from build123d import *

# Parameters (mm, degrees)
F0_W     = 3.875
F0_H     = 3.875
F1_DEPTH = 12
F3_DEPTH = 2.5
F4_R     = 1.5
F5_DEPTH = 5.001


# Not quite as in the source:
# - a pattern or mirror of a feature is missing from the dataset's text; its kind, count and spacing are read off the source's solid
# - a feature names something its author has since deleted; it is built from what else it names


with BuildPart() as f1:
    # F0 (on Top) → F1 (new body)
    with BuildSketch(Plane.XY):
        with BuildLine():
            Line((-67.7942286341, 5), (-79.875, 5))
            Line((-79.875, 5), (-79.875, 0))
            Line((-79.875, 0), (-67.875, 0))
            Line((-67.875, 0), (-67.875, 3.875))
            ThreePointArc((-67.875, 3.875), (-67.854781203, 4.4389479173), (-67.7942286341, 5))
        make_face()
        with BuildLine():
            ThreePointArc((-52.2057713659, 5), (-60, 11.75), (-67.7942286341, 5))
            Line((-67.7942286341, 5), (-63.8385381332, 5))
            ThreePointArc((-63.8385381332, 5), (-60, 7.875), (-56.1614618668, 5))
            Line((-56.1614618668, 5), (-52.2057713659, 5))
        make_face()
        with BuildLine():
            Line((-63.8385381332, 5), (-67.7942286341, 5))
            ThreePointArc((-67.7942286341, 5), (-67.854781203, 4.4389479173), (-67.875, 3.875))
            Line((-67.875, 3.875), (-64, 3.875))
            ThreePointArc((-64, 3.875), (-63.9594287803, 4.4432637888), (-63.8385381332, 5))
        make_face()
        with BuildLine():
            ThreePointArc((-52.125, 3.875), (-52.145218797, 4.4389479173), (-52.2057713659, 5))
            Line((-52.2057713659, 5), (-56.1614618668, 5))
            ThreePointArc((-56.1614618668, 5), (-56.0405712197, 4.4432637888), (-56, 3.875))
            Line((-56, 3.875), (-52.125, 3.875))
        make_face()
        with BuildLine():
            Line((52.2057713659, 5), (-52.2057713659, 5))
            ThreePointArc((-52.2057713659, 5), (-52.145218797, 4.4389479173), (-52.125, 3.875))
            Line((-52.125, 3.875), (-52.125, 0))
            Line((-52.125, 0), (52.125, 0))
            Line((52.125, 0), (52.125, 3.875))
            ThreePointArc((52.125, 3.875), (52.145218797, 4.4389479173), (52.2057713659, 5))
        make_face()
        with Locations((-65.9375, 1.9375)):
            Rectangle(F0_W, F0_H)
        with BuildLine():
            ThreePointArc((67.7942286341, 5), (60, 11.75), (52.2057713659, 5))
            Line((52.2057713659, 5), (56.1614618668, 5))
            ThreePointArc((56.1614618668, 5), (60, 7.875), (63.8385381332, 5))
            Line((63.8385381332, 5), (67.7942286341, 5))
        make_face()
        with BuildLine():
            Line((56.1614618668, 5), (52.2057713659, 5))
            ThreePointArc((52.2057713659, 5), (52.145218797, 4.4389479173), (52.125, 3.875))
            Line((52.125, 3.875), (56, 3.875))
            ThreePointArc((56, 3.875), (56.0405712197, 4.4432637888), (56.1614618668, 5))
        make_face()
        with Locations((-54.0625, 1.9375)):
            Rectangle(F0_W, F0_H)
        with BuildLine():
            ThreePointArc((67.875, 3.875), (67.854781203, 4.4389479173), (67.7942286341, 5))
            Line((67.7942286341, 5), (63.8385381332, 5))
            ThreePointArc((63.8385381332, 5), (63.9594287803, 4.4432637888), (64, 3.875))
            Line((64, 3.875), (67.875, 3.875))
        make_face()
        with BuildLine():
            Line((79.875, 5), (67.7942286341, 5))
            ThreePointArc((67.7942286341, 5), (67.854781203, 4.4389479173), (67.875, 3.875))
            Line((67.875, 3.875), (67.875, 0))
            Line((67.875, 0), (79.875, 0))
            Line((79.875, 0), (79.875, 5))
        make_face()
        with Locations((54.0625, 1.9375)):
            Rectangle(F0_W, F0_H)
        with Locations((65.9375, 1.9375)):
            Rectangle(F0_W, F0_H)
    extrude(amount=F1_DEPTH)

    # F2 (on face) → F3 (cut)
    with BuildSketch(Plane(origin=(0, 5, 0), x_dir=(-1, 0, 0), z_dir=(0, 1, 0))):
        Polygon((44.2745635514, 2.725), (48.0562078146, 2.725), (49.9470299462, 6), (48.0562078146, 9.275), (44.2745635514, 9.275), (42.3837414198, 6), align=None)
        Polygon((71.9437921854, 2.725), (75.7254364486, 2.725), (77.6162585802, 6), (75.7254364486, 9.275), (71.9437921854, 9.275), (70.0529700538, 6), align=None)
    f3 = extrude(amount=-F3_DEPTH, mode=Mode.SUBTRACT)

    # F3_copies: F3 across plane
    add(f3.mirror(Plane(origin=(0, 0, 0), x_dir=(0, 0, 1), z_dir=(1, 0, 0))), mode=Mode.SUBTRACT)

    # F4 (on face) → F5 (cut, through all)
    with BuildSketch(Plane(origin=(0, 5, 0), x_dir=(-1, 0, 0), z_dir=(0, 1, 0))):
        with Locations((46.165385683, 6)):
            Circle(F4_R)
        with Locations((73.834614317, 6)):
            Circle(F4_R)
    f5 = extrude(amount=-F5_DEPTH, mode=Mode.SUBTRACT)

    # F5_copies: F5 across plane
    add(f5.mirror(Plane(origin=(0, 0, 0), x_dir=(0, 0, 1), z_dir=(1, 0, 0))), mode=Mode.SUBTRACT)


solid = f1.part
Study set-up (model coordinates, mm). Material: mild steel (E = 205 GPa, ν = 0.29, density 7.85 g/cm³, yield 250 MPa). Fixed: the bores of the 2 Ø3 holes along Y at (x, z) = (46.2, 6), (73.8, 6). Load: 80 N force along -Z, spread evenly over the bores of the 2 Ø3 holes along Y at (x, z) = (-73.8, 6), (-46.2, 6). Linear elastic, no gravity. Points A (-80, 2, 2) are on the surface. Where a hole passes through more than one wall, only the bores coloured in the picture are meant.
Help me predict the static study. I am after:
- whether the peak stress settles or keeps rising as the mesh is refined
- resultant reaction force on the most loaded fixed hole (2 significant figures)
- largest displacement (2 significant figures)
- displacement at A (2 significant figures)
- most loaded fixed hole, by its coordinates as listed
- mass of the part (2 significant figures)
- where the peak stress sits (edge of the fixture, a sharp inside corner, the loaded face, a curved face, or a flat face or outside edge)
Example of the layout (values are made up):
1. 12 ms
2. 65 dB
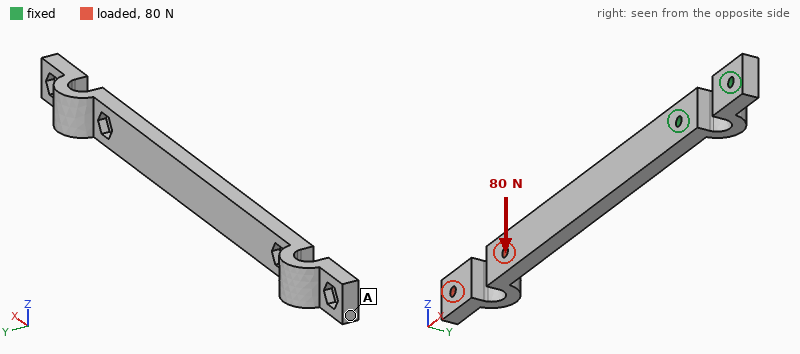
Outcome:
1. keeps rising
2. 240 N
3. 0.39 mm
4. 0.39 mm
5. (46.2, 6)
6. 76 g
7. edge of the fixture
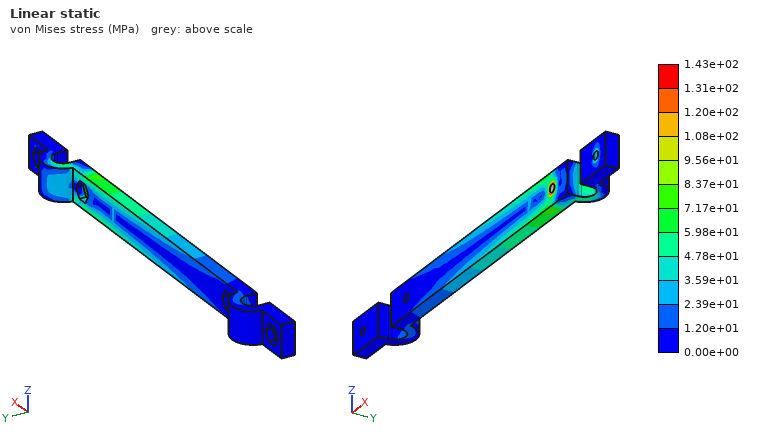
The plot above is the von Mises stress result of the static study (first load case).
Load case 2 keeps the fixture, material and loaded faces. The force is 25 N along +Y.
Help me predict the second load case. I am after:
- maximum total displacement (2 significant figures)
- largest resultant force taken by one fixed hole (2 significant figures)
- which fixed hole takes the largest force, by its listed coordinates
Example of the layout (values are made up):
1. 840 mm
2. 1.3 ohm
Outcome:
1. 0.58 mm
2. 110 N
3. (46.2, 6)
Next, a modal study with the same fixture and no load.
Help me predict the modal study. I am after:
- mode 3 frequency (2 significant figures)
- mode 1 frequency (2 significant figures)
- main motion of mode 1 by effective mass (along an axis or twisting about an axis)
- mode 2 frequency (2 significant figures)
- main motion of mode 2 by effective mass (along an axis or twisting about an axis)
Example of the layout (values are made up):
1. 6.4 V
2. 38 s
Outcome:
1. 1500 Hz
2. 240 Hz
3. along Y
4. 510 Hz
5. along Z
